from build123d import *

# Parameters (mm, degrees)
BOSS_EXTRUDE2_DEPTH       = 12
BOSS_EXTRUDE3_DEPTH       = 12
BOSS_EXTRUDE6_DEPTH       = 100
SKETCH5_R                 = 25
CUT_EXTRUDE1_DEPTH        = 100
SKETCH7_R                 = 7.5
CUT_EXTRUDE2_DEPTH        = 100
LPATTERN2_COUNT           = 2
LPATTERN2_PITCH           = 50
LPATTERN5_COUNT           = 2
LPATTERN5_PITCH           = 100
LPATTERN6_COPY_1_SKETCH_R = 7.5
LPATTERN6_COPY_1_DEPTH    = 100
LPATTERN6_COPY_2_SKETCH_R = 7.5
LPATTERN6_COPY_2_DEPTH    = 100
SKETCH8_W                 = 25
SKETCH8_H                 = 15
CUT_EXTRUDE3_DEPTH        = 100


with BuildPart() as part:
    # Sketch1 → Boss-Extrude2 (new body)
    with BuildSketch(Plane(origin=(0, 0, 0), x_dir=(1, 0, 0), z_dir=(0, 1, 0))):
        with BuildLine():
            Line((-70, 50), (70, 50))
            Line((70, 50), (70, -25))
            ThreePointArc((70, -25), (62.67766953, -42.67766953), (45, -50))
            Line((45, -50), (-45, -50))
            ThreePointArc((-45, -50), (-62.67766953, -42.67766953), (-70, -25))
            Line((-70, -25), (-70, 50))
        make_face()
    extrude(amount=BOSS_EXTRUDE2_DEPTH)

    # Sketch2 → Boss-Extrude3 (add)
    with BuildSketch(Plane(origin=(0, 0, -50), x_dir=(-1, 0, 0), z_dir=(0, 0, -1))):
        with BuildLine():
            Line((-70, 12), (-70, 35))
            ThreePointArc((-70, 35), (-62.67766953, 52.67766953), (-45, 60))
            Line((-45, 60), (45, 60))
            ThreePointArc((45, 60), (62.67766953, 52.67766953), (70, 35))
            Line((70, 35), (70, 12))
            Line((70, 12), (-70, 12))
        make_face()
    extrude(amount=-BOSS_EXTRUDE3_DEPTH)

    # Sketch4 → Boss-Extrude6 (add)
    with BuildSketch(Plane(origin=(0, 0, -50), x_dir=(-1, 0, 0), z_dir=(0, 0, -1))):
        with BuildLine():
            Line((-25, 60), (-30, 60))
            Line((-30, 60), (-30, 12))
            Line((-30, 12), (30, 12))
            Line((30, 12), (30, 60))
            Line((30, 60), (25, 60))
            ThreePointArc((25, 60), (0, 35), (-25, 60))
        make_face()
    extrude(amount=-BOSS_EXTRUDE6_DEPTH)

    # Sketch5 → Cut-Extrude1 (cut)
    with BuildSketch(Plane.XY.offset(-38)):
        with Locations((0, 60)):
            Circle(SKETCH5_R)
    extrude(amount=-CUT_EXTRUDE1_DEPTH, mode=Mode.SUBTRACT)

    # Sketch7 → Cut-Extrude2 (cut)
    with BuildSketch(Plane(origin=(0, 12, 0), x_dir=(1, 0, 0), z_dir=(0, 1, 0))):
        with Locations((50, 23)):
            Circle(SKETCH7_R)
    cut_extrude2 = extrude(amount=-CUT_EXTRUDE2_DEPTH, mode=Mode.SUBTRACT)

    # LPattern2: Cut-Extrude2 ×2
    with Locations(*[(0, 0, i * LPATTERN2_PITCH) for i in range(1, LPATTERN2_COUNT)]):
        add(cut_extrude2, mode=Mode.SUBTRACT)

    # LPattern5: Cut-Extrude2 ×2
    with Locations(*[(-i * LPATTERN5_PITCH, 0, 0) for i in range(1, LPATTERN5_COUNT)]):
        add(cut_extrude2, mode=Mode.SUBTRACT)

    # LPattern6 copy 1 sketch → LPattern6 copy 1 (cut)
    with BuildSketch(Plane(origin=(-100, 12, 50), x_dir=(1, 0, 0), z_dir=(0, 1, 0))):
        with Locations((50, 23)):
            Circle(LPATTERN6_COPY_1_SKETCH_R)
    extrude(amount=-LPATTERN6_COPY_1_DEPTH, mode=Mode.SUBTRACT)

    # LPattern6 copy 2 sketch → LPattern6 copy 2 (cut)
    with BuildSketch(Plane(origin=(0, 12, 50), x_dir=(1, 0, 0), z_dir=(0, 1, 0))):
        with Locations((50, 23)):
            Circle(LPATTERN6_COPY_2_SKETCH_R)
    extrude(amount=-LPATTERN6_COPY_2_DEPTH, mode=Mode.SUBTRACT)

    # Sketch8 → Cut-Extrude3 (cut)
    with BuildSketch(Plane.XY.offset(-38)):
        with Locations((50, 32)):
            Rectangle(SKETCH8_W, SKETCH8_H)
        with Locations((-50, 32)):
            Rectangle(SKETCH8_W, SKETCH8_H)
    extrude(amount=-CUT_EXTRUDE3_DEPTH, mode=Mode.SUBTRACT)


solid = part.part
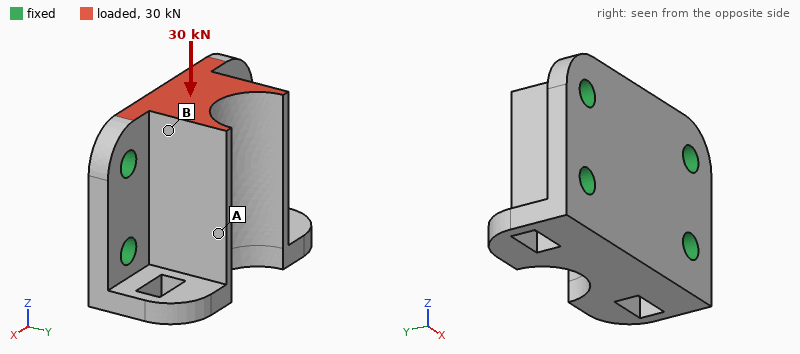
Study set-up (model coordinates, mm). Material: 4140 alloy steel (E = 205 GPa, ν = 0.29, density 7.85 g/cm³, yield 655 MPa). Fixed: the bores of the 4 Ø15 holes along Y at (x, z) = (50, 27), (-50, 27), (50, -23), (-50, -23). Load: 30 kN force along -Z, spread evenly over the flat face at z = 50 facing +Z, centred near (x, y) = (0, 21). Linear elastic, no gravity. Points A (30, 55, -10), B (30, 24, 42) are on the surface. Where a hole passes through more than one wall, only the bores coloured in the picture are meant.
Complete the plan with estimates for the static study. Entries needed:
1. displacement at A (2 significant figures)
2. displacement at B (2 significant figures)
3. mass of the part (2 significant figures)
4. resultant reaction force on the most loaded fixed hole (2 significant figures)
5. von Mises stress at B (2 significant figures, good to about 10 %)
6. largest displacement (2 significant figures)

14 µm
12 µm
3.0 kg
9.2 kN
14 MPa
20 µm
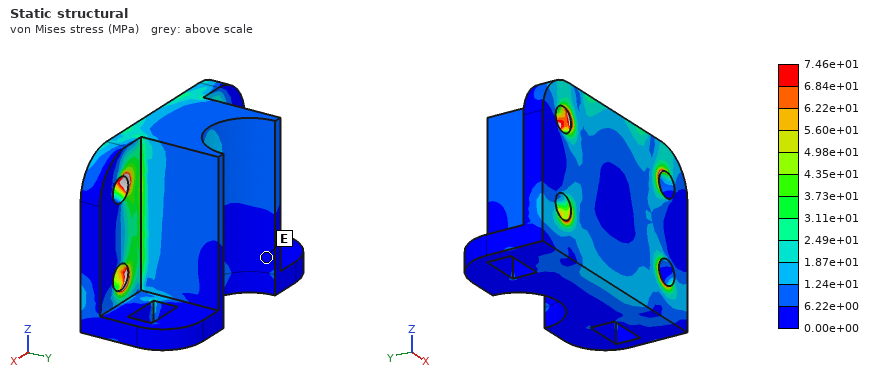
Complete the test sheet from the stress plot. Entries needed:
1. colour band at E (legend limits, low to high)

0.00e+00 to 6.22e+00 MPa
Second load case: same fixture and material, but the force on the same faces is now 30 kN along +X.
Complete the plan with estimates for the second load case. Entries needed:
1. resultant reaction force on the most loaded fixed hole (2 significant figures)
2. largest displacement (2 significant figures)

14 kN
31 µm
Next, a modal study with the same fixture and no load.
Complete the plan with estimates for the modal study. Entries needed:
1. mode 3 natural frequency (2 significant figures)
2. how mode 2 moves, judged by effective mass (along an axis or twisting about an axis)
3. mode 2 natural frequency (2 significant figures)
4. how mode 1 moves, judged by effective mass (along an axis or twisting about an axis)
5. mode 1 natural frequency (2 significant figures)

6500 Hz
along Y
5900 Hz
along Z
4200 Hz
